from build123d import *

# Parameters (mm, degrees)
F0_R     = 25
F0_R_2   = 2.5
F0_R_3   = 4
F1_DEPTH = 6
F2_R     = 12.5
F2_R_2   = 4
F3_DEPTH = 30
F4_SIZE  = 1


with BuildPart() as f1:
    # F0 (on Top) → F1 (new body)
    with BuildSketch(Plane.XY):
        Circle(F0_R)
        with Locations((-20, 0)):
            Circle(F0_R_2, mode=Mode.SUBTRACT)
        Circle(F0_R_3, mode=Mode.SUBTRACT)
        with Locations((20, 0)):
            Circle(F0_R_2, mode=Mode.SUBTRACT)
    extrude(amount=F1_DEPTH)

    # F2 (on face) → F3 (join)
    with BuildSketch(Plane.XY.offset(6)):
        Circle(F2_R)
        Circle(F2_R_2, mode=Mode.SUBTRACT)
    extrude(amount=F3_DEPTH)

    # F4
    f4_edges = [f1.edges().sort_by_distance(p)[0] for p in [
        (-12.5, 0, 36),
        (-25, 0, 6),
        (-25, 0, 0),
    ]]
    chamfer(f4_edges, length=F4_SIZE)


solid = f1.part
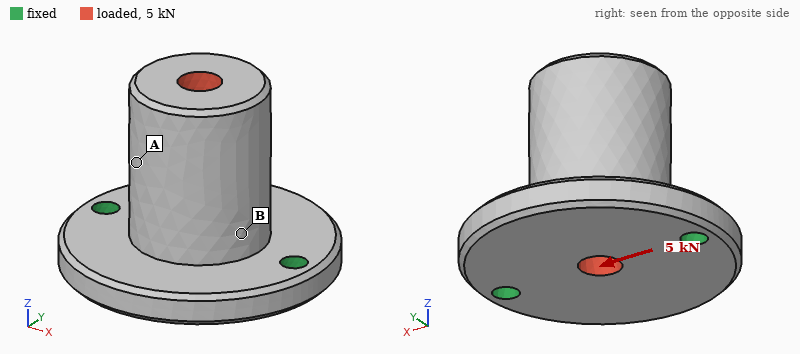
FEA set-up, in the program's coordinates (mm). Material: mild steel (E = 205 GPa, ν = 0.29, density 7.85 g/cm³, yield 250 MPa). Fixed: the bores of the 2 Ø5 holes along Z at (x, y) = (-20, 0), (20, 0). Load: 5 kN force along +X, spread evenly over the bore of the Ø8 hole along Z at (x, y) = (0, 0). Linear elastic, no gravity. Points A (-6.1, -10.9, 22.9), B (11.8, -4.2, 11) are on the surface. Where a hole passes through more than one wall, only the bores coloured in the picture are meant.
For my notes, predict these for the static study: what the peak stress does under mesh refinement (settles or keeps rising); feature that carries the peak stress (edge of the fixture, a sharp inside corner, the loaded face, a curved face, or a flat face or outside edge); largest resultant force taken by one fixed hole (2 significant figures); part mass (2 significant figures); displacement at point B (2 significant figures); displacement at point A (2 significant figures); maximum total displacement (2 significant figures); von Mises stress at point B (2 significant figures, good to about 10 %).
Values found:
keeps rising
edge of the fixture
3.4 kN
190 g
7.0 µm
12 µm
19 µm
30 MPa
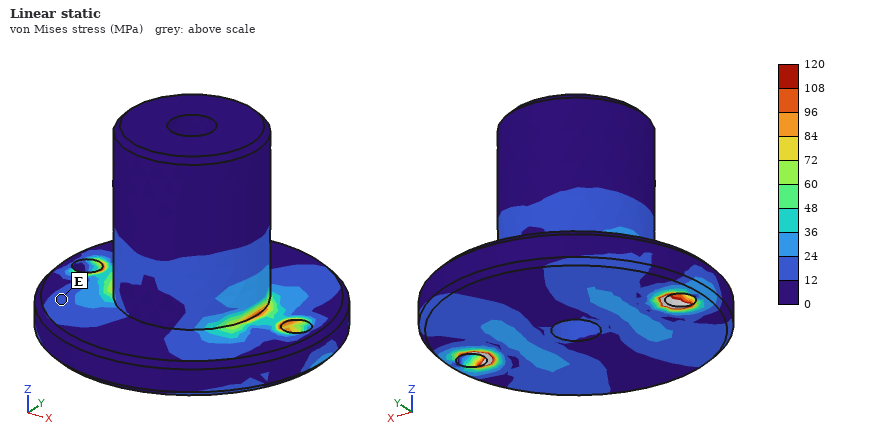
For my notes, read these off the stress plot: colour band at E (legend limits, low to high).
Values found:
12 to 24 MPa
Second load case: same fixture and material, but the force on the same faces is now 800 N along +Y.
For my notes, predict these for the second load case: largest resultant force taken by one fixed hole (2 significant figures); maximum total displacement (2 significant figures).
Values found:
400 N
16 µm
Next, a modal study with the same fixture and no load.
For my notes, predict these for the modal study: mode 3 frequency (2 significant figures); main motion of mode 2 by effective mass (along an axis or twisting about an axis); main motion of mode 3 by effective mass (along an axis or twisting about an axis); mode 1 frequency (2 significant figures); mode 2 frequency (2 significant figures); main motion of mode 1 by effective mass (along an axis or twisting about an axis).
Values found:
9700 Hz
along X
along Z
3400 Hz
8500 Hz
along Y
